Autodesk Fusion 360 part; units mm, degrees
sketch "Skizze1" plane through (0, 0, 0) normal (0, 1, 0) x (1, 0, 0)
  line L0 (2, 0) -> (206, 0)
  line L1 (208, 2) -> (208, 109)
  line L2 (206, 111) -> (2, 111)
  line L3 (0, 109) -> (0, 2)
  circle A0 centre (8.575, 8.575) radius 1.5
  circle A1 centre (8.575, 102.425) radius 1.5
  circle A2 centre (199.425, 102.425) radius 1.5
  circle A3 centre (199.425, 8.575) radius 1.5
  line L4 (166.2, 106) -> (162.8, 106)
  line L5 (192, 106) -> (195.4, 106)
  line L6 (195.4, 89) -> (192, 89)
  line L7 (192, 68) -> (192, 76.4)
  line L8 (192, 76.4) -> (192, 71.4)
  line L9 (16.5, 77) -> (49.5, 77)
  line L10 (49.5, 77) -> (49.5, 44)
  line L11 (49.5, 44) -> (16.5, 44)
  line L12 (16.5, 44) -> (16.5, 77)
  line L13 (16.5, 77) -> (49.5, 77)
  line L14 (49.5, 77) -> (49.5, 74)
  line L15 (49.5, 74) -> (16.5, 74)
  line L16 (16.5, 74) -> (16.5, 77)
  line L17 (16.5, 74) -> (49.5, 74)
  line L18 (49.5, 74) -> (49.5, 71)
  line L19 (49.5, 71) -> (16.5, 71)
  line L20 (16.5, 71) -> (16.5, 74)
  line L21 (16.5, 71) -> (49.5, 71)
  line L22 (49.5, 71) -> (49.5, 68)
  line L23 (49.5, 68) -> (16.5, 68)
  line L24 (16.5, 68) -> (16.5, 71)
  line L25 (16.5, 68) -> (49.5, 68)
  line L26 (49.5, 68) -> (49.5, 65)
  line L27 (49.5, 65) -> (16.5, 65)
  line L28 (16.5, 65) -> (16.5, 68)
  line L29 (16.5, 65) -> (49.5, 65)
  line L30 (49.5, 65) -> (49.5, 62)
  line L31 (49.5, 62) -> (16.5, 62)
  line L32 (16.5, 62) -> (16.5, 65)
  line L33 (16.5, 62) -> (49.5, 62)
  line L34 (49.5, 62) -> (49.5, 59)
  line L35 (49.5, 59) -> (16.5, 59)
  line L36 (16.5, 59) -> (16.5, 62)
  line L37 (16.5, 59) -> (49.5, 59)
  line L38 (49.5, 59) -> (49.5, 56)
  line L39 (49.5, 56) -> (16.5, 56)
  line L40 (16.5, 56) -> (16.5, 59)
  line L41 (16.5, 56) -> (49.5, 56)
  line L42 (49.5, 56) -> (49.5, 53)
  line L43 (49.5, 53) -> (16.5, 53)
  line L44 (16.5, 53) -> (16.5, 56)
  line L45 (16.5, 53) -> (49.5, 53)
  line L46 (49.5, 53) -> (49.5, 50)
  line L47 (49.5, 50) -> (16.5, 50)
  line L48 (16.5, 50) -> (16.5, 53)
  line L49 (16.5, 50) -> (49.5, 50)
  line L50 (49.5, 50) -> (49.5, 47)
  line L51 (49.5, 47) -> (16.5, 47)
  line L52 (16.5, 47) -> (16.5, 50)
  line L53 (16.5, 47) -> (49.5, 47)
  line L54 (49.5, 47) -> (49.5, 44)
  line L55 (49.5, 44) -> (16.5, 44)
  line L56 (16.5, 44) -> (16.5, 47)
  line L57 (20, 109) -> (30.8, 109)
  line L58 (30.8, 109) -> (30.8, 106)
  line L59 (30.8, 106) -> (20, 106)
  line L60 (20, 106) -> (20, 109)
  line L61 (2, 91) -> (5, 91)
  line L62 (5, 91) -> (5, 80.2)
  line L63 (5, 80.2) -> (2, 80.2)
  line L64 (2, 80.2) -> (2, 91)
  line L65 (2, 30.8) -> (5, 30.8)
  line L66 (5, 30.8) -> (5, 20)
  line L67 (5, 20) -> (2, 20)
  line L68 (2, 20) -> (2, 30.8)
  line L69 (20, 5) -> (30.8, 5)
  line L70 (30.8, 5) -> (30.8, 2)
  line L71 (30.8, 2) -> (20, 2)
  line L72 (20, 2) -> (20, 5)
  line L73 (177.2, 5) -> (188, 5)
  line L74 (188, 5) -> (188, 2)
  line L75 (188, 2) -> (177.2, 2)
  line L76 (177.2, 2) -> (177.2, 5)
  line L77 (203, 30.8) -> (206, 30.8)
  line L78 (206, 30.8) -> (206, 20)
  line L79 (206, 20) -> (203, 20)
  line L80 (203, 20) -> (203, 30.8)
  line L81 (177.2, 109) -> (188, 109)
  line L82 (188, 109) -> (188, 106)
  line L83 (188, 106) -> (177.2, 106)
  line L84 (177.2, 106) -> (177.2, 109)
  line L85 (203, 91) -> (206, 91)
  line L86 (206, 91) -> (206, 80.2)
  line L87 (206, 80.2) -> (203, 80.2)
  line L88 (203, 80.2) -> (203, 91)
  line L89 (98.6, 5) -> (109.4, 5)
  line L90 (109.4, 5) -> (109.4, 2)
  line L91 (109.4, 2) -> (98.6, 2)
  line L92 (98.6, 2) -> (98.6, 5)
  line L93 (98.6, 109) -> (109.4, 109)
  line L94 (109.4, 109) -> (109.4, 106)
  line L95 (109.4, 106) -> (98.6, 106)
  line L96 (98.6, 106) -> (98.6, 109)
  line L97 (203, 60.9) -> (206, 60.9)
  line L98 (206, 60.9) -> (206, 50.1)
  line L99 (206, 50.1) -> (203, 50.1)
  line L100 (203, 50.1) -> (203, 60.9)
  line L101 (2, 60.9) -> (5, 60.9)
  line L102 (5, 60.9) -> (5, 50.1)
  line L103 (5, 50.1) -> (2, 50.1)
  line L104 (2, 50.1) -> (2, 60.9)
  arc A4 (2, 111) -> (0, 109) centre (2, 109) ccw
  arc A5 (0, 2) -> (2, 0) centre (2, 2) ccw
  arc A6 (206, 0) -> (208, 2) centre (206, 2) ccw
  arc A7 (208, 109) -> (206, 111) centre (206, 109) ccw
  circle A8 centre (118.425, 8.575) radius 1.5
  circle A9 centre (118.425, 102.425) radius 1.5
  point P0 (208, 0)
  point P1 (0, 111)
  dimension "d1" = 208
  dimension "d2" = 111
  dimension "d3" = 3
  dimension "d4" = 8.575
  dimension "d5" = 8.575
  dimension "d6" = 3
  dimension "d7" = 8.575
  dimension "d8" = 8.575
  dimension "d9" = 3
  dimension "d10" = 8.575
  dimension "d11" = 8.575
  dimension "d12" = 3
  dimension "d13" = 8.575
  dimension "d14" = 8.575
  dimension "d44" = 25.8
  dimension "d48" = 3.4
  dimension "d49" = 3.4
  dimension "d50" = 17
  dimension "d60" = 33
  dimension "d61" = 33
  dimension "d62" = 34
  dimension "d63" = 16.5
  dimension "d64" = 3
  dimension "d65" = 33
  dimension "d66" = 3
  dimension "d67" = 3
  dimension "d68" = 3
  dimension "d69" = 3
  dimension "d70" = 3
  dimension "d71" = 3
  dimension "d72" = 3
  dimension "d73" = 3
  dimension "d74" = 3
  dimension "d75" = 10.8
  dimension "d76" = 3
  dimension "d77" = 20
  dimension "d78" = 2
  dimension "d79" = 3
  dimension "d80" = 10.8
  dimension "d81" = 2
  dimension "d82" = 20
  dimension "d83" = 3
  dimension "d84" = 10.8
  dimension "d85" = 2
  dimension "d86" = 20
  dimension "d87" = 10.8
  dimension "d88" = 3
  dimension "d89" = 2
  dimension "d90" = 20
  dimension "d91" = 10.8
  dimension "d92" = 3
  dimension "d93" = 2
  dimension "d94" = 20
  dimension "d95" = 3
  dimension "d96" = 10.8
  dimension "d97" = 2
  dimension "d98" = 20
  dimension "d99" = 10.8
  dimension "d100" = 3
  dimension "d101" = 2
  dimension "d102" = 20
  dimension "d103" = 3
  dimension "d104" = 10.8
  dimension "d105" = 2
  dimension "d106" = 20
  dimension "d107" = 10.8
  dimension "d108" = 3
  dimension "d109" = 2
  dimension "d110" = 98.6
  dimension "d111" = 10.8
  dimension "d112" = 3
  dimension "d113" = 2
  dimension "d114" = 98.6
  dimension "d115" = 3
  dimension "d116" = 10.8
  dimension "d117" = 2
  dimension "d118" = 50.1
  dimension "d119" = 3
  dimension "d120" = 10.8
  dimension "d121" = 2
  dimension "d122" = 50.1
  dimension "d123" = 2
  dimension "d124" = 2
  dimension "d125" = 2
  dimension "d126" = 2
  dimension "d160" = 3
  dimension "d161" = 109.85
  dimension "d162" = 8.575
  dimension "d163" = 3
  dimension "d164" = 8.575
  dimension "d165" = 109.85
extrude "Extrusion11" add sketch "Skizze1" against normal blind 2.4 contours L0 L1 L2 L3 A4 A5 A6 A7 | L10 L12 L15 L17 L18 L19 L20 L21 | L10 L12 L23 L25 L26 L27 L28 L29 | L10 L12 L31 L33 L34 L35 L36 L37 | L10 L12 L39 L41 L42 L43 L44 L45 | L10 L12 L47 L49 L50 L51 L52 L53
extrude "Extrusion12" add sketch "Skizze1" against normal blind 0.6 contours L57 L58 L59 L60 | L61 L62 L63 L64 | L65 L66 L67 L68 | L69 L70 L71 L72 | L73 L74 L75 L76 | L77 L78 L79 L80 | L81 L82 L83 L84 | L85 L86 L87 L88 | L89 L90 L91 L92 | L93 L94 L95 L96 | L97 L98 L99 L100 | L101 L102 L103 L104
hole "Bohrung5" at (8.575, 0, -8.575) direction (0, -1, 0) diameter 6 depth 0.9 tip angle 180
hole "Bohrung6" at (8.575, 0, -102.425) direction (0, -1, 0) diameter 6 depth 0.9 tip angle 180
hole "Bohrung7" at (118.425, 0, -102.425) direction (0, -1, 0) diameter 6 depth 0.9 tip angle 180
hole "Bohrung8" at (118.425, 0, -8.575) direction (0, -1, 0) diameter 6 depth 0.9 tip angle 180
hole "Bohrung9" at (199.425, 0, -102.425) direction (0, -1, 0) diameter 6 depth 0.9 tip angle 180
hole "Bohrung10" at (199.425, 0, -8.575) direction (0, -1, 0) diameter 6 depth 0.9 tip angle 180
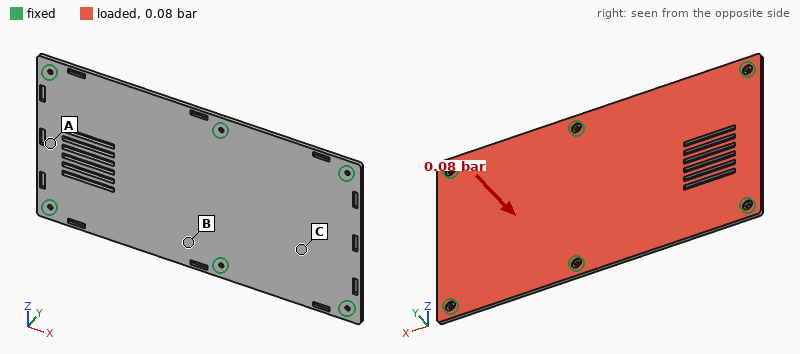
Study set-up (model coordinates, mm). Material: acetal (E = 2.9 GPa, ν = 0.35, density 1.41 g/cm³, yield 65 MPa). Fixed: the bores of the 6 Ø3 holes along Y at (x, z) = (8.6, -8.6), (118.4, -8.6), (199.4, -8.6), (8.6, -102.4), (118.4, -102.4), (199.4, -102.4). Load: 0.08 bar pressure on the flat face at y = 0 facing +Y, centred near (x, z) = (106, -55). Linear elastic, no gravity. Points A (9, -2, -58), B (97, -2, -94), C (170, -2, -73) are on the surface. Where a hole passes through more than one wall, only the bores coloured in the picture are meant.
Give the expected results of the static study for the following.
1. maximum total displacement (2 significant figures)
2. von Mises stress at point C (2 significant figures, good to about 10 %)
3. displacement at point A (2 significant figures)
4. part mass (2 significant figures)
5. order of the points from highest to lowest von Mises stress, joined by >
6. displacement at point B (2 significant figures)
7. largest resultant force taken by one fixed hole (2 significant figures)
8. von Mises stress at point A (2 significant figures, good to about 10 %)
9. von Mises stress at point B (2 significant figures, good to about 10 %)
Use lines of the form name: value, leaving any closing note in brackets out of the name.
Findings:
maximum total displacement: 2.4 mm
von Mises stress at point C: 3.0 MPa
displacement at point A: 1.2 mm
part mass: 75 g
order of the points from highest to lowest von Mises stress, joined by >: A > C > B
displacement at point B: 0.89 mm
largest resultant force taken by one fixed hole: 75 N
von Mises stress at point A: 6.9 MPa
von Mises stress at point B: 1.7 MPa
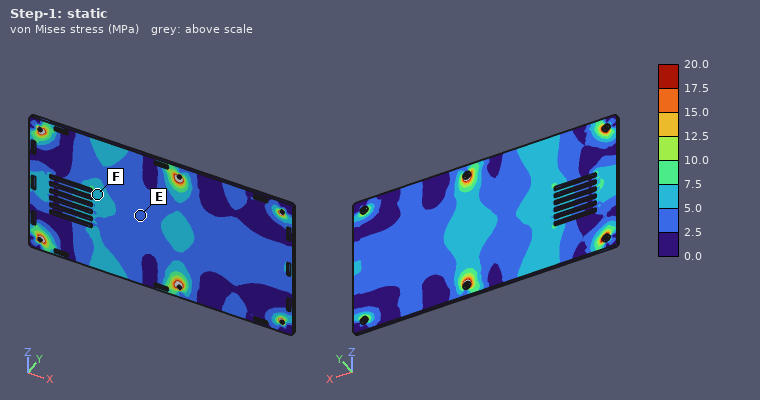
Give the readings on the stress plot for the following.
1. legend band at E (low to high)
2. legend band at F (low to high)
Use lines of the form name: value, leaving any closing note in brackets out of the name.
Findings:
legend band at E: 2.5 to 5.0 MPa
legend band at F: 5.0 to 7.5 MPa
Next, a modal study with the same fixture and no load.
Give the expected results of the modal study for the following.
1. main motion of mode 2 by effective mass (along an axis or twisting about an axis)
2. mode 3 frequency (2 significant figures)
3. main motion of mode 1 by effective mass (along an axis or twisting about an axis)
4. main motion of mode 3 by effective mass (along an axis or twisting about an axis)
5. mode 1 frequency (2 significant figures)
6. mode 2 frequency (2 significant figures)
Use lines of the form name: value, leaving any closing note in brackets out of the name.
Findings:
main motion of mode 2 by effective mass: along Y
mode 3 frequency: 300 Hz
main motion of mode 1 by effective mass: along Y
main motion of mode 3 by effective mass: twisting about X
mode 1 frequency: 190 Hz
mode 2 frequency: 270 Hz
